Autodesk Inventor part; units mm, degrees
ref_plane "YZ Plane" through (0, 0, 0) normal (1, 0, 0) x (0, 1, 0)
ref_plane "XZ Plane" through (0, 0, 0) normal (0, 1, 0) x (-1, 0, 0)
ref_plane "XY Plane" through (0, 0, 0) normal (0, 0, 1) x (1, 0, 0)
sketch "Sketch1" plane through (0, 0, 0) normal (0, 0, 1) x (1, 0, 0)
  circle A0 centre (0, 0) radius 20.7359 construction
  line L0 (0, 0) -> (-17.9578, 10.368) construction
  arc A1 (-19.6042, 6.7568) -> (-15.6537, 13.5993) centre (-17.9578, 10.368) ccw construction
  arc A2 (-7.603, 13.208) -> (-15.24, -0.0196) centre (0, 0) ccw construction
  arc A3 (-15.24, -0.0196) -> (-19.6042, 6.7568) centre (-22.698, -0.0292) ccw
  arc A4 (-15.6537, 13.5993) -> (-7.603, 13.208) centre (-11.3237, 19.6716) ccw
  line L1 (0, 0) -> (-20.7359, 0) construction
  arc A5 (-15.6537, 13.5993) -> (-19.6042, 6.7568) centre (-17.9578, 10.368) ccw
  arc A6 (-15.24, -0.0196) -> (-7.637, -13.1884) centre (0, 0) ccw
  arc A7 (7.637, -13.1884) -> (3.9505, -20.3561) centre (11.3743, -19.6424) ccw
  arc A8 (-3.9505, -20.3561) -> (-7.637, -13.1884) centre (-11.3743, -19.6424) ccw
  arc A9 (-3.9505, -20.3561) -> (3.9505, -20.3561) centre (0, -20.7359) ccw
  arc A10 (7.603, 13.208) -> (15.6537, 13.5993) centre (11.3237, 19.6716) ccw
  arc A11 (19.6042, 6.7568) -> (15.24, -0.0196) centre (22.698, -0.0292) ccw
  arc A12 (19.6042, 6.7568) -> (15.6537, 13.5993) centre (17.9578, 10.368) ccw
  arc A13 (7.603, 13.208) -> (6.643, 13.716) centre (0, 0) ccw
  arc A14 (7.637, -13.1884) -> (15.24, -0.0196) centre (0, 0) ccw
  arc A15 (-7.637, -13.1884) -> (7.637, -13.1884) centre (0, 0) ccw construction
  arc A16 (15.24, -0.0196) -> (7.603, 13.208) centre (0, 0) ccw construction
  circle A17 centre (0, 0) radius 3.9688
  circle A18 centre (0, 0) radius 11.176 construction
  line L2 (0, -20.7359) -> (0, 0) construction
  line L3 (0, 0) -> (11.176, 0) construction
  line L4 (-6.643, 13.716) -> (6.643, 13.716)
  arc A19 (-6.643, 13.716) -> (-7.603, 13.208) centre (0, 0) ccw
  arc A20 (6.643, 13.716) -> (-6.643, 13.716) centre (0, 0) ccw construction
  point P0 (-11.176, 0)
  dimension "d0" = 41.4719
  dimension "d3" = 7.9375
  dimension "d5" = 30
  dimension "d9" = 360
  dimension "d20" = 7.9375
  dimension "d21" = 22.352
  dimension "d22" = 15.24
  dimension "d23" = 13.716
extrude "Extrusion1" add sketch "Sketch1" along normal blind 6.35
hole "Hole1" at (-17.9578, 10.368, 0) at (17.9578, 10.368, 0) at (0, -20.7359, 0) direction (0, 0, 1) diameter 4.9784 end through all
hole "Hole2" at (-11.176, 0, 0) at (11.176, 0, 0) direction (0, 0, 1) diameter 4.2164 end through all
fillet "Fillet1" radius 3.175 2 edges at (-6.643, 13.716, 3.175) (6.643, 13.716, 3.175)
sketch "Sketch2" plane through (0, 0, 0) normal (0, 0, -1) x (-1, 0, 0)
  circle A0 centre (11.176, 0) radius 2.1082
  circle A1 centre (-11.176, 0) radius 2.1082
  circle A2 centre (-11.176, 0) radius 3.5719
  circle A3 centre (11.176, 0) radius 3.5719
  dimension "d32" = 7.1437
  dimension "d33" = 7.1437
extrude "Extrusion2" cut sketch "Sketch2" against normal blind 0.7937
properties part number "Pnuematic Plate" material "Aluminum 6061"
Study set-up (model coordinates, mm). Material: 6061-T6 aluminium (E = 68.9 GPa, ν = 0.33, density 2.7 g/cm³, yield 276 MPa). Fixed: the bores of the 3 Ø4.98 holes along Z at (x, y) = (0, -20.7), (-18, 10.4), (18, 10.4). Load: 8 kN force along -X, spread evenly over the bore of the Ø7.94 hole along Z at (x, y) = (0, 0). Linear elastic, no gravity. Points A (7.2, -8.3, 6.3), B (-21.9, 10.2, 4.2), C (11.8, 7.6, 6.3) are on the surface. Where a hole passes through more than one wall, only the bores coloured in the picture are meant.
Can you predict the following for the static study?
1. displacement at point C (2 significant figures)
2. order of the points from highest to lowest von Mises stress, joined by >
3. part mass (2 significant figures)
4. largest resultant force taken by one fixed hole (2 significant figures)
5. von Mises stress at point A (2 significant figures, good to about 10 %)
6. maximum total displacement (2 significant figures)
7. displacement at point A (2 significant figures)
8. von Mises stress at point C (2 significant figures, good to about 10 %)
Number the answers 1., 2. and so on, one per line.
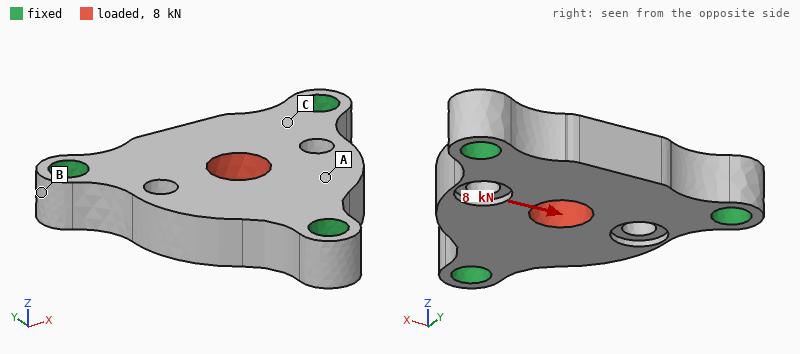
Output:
1. 5.2 µm
2. C > A > B
3. 14 g
4. 3.3 kN
5. 27 MPa
6. 25 µm
7. 19 µm
8. 59 MPa
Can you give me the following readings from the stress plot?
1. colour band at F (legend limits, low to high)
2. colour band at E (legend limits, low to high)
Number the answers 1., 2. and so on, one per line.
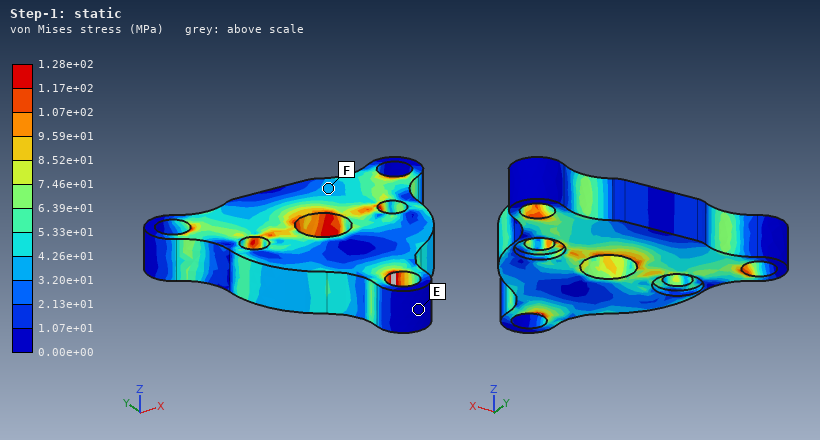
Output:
1. 3.20e+01 to 4.26e+01 MPa
2. 0.00e+00 to 1.07e+01 MPa
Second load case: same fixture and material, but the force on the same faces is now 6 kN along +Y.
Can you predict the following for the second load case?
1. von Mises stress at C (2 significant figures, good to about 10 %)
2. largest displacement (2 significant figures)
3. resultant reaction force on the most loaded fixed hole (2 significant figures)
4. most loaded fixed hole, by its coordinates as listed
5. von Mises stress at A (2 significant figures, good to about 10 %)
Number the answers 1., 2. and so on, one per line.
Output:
1. 35 MPa
2. 19 µm
3. 3.2 kN
4. (0, -20.7)
5. 27 MPa
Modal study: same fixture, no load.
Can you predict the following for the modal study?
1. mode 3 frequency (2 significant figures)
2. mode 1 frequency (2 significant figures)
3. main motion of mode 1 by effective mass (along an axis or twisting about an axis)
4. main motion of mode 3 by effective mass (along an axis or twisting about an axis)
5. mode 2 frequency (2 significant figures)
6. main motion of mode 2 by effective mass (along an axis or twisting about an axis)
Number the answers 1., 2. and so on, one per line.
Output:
1. 27 kHz
2. 20 kHz
3. along Z
4. twisting about X
5. 24 kHz
6. twisting about Y
